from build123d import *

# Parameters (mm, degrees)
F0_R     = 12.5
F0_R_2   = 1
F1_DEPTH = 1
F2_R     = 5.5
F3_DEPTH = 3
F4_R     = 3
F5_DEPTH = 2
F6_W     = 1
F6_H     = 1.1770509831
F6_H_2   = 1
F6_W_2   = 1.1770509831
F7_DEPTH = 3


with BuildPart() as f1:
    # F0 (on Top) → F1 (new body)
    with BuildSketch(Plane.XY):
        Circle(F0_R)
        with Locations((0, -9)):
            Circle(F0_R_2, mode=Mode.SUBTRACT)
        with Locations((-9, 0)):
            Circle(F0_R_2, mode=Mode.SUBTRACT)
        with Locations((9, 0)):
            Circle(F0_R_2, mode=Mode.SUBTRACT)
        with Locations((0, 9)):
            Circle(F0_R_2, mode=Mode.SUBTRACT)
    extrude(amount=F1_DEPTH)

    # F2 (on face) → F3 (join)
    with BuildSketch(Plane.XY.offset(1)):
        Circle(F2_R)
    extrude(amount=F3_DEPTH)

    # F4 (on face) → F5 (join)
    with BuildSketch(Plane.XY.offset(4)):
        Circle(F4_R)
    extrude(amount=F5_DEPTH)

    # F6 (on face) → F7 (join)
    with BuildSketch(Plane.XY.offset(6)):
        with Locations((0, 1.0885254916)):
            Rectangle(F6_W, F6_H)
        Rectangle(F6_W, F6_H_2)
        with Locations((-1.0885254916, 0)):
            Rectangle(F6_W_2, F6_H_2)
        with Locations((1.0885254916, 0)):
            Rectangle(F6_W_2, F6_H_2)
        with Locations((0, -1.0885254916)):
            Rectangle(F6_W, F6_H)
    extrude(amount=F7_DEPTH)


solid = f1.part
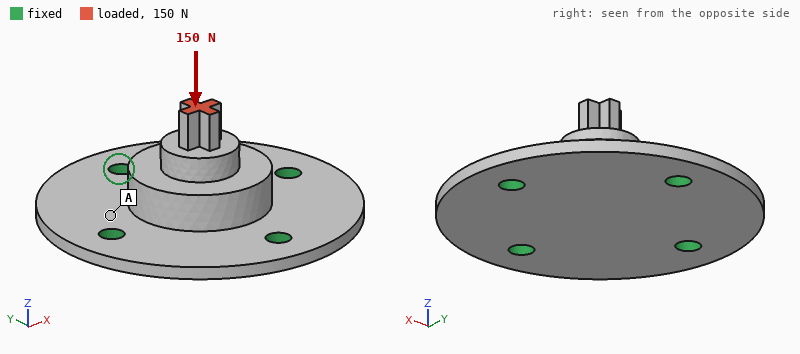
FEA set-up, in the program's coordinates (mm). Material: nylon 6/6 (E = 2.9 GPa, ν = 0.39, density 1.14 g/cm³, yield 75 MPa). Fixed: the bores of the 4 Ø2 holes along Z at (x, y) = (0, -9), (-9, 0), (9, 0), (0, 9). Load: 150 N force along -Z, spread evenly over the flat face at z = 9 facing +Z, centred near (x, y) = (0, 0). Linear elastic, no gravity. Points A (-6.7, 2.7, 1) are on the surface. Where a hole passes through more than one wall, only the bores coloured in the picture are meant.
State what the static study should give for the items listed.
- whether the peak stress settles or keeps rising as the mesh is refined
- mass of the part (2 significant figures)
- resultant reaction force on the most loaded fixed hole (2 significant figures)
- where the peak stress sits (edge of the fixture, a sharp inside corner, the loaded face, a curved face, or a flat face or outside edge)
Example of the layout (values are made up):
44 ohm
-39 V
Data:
keeps rising
0.95 g
42 N
edge of the fixture
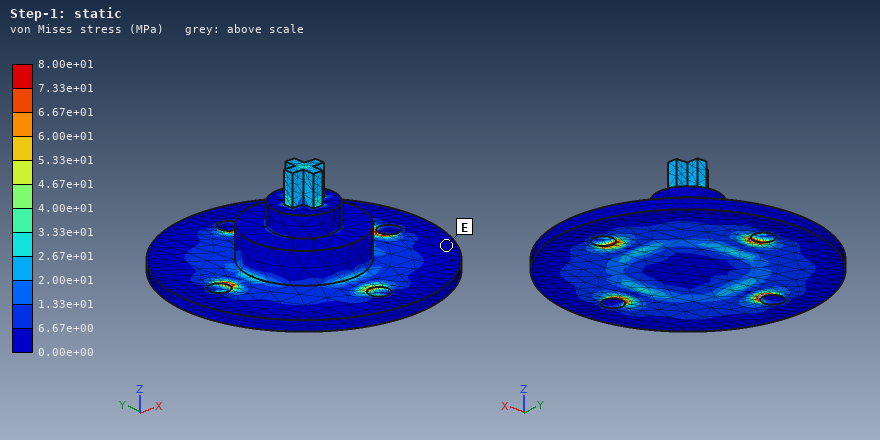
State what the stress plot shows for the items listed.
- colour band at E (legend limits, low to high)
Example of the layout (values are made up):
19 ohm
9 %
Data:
0.00e+00 to 6.67e+00 MPa
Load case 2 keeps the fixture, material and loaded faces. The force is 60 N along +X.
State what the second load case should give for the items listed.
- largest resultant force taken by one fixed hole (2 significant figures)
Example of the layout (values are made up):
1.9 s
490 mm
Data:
41 N
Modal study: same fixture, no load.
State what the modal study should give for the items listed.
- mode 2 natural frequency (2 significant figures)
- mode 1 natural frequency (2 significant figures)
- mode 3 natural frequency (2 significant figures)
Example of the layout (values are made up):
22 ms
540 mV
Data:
7500 Hz
7400 Hz
7500 Hz
